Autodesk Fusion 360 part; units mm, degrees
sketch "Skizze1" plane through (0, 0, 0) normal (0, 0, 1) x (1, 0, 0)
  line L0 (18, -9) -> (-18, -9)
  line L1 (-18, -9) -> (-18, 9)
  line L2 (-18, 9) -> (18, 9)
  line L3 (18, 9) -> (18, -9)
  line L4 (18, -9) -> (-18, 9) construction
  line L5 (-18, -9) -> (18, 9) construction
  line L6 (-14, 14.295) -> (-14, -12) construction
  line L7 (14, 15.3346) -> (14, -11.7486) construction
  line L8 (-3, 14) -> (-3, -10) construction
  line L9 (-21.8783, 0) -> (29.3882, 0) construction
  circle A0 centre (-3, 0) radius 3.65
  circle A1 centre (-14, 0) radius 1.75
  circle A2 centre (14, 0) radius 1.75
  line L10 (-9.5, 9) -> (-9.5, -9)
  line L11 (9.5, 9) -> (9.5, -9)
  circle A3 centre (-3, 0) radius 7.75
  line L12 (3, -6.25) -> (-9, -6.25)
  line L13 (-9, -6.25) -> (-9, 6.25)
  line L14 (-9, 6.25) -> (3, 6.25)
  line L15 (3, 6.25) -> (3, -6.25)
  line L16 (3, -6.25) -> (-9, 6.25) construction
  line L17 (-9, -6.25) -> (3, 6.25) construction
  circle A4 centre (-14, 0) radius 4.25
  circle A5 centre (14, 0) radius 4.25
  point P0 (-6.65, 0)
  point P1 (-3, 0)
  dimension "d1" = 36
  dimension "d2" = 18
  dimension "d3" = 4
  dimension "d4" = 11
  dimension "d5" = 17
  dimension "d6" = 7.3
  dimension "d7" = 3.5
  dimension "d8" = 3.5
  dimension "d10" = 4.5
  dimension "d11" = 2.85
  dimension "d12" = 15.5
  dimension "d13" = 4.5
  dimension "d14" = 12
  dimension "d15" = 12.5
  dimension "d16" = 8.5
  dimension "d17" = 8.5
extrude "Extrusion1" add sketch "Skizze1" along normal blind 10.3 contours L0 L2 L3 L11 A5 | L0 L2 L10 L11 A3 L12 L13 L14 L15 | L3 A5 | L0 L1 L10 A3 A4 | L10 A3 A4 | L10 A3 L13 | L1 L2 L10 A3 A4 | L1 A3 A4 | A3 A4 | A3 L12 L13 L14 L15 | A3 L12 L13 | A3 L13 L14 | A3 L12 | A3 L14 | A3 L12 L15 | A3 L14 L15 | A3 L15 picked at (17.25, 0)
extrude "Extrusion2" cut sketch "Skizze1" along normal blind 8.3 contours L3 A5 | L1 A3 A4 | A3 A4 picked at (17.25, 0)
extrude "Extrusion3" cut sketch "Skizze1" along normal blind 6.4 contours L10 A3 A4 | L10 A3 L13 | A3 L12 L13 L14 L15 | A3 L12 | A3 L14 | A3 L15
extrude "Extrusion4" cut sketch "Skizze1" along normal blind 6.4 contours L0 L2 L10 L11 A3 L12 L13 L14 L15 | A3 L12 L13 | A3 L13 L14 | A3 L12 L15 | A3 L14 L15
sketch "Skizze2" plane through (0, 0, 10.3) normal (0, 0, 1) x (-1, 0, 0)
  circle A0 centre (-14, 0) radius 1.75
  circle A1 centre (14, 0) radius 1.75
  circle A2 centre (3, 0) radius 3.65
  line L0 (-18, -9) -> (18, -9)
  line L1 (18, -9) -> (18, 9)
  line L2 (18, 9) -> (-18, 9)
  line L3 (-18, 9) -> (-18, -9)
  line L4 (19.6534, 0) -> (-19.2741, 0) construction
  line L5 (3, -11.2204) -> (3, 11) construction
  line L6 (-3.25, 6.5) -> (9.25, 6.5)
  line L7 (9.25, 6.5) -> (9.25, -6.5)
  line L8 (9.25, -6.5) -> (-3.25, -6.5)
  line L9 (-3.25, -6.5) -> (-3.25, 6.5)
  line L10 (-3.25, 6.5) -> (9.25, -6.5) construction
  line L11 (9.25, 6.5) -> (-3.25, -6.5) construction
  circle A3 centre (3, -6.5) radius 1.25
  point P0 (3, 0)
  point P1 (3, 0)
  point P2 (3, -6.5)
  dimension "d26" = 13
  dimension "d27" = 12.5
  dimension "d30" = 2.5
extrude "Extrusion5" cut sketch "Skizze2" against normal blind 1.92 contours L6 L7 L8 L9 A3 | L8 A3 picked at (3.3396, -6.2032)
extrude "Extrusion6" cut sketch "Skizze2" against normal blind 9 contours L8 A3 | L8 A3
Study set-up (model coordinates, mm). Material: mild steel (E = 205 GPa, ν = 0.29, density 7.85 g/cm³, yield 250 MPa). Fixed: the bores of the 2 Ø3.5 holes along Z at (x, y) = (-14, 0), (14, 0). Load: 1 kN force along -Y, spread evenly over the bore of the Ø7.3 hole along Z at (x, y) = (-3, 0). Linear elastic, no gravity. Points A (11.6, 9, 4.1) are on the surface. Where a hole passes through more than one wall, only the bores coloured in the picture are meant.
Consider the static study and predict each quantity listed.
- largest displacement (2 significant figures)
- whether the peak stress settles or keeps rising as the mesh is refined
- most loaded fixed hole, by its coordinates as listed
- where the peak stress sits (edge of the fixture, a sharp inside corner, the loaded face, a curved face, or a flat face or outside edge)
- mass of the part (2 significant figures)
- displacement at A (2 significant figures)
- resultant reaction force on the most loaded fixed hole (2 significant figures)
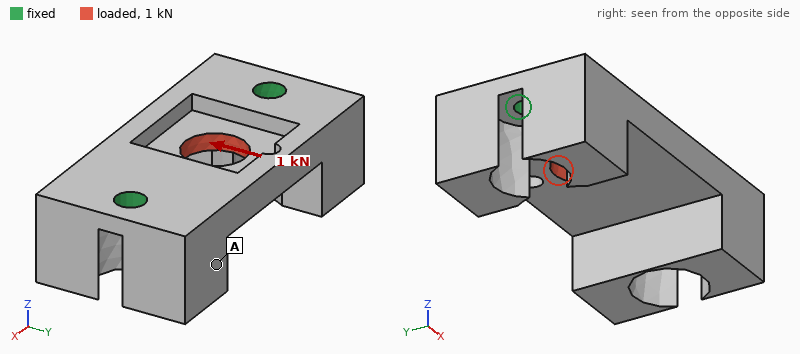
11 µm
keeps rising
(-14, 0)
edge of the fixture
24 g
6.0 µm
590 N
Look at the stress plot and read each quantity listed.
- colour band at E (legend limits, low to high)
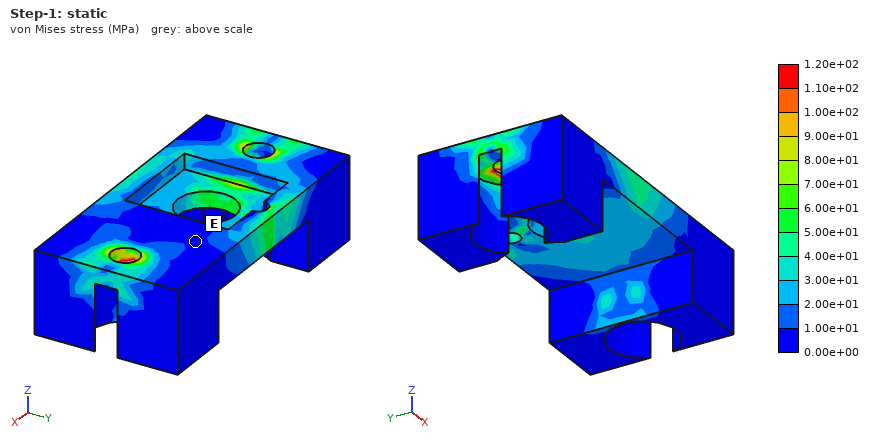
0.00e+00 to 1.00e+01 MPa
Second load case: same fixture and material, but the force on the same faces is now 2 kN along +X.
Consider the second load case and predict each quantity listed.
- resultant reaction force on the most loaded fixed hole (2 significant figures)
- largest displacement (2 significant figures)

1.1 kN
5.4 µm
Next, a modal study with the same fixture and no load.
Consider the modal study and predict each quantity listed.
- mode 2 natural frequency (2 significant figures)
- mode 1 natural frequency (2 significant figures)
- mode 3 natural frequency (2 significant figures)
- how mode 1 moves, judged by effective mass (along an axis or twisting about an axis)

12 kHz
8200 Hz
12 kHz
along Y
